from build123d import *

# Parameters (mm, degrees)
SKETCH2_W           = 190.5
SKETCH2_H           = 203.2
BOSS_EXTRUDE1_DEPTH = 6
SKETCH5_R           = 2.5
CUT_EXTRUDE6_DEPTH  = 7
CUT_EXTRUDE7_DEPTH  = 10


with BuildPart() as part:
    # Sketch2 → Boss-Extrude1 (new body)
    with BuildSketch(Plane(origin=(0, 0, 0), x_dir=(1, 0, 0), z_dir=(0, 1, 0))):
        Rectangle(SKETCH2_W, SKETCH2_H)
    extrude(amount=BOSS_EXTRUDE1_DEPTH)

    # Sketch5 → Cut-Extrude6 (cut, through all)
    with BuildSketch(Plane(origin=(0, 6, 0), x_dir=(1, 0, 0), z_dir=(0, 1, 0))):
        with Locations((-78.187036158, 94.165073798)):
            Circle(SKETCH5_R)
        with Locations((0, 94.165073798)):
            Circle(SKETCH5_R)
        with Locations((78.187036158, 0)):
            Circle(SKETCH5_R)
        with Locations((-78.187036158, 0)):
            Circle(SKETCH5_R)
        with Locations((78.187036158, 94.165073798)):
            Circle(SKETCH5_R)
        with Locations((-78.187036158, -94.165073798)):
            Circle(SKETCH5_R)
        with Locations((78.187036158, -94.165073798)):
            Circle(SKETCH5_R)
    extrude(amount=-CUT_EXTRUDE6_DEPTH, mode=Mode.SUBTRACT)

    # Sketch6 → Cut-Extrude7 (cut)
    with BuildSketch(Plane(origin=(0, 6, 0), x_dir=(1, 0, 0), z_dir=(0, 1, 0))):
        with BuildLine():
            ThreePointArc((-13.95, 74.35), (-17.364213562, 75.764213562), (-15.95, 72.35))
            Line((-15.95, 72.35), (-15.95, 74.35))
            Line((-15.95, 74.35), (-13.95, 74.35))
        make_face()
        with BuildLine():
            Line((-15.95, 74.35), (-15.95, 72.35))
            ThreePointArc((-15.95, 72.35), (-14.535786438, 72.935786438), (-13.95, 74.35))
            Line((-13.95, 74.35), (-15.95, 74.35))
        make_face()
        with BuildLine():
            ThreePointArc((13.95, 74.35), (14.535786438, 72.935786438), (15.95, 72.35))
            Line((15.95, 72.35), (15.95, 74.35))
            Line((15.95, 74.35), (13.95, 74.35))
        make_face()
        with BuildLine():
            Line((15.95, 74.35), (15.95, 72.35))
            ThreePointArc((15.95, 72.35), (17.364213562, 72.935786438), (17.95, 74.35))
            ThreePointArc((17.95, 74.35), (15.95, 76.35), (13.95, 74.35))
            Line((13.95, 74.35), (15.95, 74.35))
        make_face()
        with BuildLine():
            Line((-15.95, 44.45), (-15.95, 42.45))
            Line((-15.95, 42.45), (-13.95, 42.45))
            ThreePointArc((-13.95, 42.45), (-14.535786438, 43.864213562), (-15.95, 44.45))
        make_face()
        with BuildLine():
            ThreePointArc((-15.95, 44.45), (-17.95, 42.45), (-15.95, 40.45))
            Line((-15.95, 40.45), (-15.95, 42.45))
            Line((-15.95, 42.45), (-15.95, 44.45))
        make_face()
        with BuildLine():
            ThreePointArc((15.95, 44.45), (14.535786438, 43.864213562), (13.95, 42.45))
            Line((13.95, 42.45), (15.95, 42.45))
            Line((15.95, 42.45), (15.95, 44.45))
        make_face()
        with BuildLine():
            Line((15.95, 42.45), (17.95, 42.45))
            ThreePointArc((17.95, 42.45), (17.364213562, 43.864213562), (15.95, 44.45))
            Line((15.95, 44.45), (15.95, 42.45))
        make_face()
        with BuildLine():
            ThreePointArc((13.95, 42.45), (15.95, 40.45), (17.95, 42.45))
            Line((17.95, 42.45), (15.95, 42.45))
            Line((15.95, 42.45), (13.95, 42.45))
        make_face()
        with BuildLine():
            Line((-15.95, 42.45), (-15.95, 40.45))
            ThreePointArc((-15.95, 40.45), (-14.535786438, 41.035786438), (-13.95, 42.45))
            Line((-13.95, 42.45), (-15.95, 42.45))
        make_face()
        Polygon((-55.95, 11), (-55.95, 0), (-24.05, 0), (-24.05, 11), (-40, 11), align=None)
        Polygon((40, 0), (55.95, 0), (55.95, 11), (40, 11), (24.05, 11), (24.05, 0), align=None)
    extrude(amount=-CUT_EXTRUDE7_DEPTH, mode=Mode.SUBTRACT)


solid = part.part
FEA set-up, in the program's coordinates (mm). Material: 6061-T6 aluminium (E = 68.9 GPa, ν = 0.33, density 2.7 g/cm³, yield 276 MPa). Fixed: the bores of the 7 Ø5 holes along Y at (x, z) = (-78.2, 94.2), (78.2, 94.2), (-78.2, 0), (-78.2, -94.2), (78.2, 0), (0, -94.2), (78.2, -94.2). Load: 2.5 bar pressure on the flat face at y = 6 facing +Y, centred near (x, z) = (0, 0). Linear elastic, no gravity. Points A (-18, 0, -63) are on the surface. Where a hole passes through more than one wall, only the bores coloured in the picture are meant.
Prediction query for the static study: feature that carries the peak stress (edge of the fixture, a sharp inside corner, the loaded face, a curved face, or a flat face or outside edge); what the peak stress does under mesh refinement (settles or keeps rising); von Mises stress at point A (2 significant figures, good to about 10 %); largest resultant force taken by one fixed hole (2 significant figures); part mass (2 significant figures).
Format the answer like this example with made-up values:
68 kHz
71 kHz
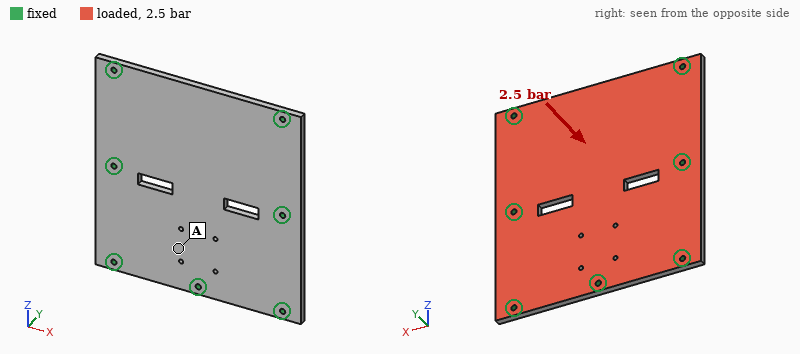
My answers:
edge of the fixture
keeps rising
20 MPa
2.1 kN
610 g
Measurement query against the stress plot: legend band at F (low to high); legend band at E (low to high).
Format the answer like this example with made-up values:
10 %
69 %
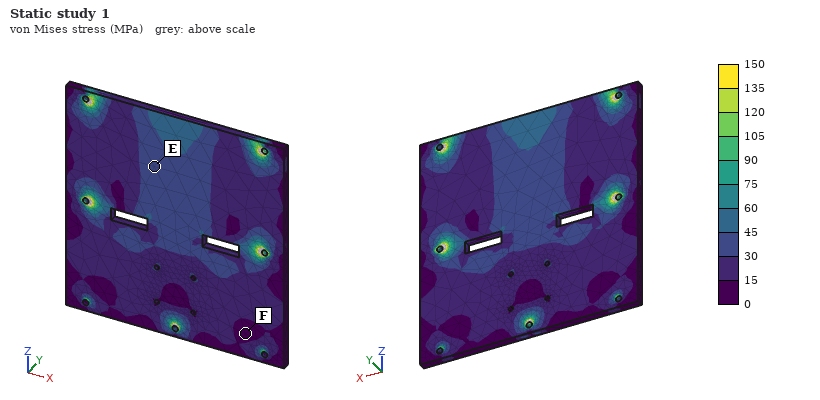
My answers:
0 to 15 MPa
30 to 45 MPa
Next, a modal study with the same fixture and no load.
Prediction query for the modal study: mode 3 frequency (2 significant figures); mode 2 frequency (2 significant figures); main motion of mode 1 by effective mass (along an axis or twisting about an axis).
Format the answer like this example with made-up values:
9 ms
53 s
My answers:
2500 Hz
1700 Hz
along Y
